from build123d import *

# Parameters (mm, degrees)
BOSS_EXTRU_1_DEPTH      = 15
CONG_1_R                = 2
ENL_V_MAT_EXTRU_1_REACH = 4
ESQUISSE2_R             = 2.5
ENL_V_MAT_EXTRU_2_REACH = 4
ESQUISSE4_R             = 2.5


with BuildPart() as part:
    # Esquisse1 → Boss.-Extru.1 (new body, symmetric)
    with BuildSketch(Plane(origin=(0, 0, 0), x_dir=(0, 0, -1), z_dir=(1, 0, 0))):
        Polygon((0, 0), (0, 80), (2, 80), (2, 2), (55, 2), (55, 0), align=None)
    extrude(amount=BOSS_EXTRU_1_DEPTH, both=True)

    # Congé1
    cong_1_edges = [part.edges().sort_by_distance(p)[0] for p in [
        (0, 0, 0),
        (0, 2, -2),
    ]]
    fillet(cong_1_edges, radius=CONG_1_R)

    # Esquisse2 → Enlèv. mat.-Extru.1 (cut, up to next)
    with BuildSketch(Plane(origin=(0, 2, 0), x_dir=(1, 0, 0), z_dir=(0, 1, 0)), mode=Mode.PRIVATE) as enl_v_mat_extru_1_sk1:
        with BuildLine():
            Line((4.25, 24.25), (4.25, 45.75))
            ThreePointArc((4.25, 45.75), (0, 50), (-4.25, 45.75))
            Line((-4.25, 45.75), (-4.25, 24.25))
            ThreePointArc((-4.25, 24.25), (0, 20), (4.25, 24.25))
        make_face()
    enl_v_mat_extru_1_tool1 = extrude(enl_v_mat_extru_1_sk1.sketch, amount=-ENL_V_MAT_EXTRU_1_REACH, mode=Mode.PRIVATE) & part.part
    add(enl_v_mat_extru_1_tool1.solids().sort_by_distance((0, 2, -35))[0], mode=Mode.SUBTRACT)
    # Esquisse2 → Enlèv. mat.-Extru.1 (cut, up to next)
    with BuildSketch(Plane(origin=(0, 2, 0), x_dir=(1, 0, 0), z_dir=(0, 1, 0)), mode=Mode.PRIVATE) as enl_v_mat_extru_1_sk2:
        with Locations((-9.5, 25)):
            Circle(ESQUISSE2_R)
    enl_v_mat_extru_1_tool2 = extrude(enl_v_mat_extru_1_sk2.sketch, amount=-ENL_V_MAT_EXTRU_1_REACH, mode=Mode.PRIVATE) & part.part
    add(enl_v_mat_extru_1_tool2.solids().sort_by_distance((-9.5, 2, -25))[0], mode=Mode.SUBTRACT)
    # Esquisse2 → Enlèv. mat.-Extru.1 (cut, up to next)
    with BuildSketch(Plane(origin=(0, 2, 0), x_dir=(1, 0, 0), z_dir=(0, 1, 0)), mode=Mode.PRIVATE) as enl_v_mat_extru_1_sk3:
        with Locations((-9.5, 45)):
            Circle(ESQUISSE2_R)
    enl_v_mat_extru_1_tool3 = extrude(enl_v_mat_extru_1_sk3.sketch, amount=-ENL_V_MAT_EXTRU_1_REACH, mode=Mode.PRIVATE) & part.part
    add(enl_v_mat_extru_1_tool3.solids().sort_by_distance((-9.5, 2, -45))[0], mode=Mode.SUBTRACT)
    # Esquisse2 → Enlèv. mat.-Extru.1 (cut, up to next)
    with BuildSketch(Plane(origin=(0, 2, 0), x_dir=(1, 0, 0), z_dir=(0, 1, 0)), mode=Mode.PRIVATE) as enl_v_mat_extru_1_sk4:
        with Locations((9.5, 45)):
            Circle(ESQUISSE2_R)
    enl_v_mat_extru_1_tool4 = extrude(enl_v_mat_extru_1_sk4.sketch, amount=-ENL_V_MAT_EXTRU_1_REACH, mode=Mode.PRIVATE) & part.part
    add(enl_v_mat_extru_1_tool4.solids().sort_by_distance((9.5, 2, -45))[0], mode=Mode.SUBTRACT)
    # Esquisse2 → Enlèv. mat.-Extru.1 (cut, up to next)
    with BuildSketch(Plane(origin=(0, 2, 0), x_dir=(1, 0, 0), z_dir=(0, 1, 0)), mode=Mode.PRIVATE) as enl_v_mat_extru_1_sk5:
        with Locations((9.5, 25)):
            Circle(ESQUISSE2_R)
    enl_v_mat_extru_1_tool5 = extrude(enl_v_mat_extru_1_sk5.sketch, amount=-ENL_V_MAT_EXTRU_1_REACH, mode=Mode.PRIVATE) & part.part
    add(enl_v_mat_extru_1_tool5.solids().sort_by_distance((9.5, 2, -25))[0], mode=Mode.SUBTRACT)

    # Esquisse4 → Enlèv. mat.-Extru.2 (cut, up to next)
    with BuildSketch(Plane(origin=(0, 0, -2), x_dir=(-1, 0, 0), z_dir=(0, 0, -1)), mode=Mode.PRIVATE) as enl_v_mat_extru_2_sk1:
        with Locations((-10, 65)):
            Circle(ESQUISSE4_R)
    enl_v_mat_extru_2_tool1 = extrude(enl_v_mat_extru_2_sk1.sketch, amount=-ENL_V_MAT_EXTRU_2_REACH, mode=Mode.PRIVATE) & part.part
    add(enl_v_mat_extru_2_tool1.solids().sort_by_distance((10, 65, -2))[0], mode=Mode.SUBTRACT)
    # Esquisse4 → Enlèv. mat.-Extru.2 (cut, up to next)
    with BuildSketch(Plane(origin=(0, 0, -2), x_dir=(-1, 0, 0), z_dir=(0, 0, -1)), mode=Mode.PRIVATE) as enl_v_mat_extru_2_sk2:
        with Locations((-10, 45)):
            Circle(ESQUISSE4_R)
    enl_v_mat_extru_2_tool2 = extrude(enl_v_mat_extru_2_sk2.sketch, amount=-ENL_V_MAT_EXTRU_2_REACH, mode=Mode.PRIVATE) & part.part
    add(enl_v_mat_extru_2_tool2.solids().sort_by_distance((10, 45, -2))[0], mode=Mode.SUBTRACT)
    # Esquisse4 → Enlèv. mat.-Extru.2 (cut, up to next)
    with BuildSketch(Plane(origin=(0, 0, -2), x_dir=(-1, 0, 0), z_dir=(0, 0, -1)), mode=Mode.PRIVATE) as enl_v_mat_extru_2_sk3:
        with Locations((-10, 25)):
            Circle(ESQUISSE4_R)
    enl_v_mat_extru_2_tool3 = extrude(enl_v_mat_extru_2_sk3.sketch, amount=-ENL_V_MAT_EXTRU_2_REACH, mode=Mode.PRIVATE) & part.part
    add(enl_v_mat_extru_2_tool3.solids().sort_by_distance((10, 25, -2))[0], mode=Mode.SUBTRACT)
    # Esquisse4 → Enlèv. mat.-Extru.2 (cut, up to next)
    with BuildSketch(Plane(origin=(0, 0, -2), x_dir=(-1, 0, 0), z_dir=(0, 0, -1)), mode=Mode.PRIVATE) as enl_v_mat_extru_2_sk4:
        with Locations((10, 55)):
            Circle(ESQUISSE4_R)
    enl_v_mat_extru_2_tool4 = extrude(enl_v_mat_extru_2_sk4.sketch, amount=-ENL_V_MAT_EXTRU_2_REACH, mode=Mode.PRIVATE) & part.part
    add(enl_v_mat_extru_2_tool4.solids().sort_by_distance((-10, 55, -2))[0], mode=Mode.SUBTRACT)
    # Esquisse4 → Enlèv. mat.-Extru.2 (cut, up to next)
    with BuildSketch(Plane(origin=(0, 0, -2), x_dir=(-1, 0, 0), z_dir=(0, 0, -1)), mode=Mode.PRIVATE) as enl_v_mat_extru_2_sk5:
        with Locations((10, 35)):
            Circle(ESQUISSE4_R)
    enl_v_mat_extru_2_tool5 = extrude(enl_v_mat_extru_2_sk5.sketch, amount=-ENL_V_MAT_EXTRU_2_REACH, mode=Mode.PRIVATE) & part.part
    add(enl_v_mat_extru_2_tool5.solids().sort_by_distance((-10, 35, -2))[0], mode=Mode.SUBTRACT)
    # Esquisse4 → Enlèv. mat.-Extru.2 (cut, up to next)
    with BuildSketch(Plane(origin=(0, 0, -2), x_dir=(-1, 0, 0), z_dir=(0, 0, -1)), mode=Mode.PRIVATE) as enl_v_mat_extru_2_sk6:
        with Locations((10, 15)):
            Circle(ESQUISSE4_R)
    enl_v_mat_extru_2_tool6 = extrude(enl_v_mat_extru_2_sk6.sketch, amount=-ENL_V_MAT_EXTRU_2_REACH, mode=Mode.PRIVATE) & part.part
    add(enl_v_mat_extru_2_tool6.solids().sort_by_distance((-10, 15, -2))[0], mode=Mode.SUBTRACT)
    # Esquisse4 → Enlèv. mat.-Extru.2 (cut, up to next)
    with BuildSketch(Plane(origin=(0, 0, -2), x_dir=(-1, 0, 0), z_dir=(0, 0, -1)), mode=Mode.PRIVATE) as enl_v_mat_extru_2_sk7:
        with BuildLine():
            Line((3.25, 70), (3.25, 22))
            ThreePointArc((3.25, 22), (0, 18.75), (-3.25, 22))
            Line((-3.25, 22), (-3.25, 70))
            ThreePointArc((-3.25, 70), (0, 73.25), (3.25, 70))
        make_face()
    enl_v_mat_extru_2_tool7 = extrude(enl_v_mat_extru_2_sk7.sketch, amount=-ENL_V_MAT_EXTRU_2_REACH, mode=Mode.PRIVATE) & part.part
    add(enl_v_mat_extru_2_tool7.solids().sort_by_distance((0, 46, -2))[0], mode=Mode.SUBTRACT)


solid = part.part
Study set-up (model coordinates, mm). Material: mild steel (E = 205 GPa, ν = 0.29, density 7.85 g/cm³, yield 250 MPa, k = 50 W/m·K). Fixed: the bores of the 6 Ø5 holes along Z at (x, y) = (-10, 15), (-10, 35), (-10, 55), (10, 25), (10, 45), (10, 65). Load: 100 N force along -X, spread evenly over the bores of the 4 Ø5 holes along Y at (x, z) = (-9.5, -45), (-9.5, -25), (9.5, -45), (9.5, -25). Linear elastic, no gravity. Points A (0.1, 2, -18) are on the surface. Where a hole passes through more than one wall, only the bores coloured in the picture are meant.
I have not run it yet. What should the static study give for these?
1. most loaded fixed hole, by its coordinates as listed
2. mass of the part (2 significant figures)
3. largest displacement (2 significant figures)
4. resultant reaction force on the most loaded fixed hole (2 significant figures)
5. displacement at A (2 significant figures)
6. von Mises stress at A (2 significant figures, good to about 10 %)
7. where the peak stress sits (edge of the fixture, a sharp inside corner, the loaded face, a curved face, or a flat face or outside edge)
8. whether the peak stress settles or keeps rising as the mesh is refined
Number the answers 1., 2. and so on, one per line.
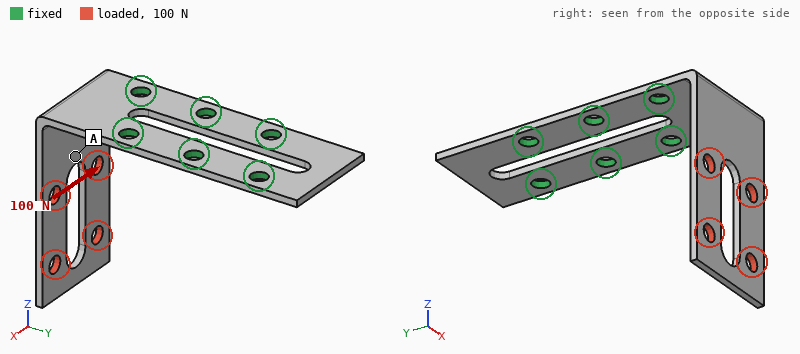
1. (-10, 15)
2. 50 g
3. 0.30 mm
4. 140 N
5. 0.092 mm
6. 19 MPa
7. edge of the fixture
8. keeps rising
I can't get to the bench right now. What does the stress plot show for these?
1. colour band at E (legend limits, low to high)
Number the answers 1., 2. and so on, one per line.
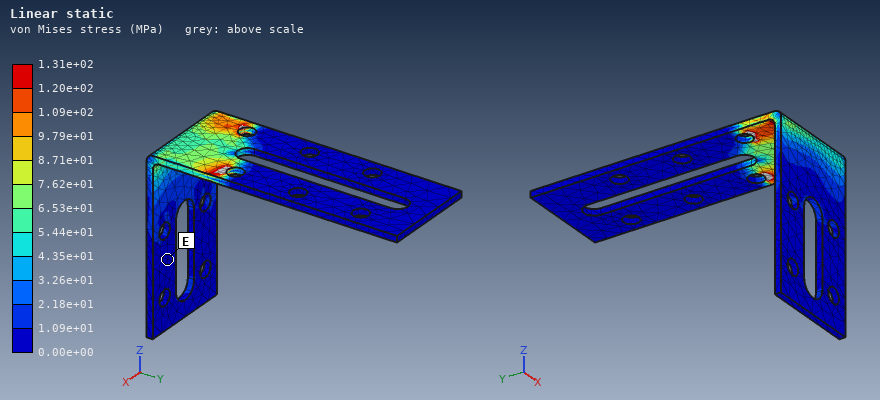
1. 0.00e+00 to 1.09e+01 MPa
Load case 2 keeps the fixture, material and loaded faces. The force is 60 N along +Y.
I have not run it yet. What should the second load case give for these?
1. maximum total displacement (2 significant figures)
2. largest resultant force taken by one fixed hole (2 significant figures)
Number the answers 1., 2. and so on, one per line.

1. 0.75 mm
2. 47 N
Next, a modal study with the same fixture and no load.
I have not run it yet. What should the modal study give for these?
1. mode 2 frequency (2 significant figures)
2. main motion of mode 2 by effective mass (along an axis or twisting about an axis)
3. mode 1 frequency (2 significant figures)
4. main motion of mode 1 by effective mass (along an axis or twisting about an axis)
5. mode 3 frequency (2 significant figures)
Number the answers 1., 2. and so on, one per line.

1. 960 Hz
2. along X
3. 450 Hz
4. along Y
5. 1900 Hz
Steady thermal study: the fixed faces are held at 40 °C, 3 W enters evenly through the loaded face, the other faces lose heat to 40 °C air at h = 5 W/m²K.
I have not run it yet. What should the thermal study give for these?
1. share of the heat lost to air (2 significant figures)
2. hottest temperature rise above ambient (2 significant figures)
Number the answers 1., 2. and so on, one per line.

1. 19 %
2. 52 K
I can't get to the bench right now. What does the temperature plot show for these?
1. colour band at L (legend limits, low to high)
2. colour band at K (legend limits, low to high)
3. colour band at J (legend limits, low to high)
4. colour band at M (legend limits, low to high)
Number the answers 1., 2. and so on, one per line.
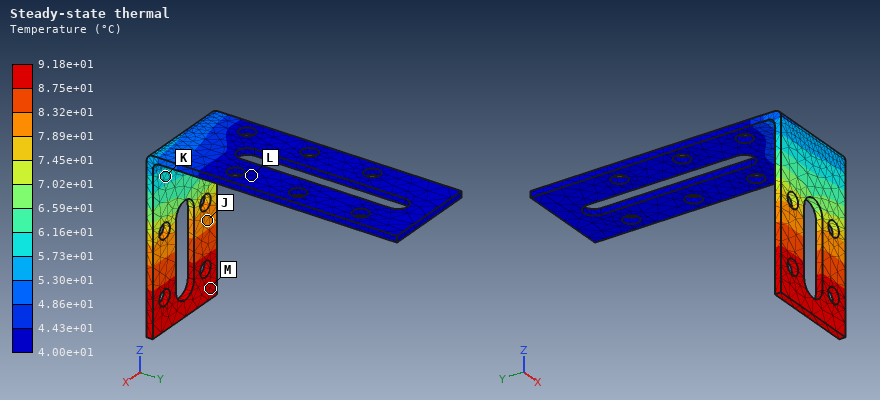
1. 4.00e+01 to 4.43e+01 °C
2. 5.73e+01 to 6.16e+01 °C
3. 7.89e+01 to 8.32e+01 °C
4. 8.75e+01 to 9.18e+01 °C
